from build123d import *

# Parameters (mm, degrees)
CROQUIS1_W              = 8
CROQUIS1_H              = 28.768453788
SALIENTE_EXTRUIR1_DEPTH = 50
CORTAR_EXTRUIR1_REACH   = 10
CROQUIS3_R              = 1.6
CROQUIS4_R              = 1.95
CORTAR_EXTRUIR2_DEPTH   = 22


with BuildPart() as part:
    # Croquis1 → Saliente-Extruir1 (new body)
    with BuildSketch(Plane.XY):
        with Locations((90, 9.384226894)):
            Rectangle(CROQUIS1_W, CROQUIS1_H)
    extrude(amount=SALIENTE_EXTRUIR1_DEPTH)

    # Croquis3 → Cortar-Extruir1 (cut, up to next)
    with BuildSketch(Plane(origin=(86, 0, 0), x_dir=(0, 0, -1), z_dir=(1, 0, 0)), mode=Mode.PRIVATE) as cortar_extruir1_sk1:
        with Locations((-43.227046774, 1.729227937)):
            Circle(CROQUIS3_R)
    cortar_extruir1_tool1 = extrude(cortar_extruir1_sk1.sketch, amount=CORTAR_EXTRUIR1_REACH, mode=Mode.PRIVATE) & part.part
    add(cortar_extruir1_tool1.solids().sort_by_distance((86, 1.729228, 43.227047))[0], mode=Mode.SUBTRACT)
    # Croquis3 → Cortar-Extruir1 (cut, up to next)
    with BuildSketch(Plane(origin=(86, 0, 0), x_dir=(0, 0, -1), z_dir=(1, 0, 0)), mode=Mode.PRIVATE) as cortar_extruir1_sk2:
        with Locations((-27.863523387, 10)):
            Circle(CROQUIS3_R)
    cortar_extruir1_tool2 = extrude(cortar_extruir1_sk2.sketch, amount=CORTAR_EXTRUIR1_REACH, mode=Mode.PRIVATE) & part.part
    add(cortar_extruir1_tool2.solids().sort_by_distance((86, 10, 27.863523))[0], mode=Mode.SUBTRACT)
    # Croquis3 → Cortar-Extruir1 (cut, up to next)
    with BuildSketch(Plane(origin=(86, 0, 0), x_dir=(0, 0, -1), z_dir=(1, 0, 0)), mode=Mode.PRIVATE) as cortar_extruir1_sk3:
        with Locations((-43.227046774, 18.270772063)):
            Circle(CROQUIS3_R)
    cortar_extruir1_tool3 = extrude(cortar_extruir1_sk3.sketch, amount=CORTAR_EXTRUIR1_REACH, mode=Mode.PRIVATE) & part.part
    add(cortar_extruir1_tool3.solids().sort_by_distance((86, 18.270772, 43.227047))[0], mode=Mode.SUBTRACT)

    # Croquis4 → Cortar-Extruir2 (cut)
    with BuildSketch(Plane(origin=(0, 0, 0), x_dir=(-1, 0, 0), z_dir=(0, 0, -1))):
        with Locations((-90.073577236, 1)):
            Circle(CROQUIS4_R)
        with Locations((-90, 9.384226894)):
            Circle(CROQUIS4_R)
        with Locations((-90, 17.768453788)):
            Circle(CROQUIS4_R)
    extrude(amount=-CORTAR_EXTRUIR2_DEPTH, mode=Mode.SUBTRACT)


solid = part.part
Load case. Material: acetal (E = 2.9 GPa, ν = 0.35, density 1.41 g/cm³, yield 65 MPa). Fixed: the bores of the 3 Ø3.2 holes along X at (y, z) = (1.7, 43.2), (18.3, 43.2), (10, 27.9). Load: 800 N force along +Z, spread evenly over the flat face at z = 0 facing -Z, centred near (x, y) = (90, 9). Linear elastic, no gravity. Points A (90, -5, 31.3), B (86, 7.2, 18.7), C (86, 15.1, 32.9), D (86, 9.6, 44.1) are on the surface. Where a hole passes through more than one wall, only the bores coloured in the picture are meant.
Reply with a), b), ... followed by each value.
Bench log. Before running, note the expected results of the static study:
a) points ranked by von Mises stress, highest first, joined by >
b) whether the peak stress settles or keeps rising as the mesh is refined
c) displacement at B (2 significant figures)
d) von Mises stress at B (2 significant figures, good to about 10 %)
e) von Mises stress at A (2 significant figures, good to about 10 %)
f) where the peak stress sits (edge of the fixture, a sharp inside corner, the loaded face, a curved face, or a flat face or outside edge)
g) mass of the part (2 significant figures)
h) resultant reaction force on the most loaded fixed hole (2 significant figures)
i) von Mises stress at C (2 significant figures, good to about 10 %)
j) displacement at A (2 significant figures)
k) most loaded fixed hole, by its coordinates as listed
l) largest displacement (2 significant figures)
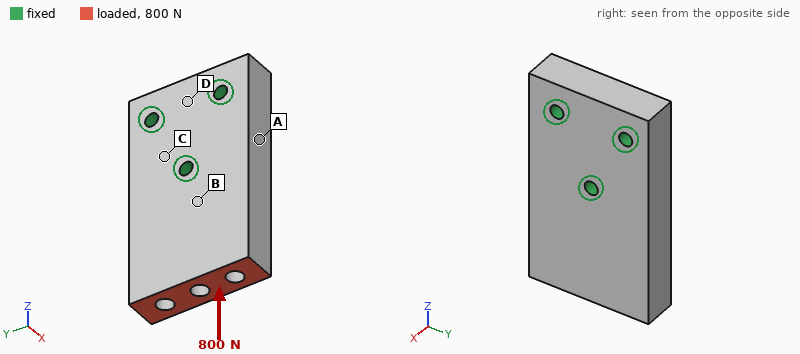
a) B > A > C > D
b) keeps rising
c) 19 µm
d) 5.2 MPa
e) 2.8 MPa
f) edge of the fixture
g) 15 g
h) 470 N
i) 1.8 MPa
j) 13 µm
k) (10, 27.9)
l) 51 µm
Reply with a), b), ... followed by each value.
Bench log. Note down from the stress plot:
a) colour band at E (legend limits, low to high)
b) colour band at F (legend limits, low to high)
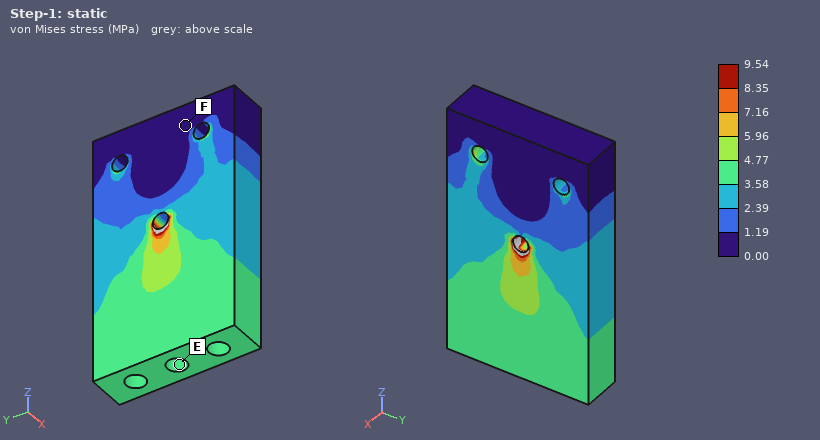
a) 3.58 to 4.77 MPa
b) 0.00 to 1.19 MPa
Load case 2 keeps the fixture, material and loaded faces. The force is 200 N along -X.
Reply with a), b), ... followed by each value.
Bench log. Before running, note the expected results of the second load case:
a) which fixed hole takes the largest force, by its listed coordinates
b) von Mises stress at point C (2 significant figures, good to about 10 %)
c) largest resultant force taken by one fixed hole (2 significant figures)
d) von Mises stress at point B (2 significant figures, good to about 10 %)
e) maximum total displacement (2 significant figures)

a) (10, 27.9)
b) 5.1 MPa
c) 380 N
d) 12 MPa
e) 0.56 mm
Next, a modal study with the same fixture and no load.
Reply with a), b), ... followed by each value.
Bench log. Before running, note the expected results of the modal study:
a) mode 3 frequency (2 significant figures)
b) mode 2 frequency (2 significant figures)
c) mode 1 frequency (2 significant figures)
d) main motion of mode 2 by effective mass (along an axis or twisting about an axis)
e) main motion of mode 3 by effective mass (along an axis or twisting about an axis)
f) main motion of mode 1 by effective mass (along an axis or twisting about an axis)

a) 3900 Hz
b) 3600 Hz
c) 2100 Hz
d) twisting about Z
e) along Y
f) along X
